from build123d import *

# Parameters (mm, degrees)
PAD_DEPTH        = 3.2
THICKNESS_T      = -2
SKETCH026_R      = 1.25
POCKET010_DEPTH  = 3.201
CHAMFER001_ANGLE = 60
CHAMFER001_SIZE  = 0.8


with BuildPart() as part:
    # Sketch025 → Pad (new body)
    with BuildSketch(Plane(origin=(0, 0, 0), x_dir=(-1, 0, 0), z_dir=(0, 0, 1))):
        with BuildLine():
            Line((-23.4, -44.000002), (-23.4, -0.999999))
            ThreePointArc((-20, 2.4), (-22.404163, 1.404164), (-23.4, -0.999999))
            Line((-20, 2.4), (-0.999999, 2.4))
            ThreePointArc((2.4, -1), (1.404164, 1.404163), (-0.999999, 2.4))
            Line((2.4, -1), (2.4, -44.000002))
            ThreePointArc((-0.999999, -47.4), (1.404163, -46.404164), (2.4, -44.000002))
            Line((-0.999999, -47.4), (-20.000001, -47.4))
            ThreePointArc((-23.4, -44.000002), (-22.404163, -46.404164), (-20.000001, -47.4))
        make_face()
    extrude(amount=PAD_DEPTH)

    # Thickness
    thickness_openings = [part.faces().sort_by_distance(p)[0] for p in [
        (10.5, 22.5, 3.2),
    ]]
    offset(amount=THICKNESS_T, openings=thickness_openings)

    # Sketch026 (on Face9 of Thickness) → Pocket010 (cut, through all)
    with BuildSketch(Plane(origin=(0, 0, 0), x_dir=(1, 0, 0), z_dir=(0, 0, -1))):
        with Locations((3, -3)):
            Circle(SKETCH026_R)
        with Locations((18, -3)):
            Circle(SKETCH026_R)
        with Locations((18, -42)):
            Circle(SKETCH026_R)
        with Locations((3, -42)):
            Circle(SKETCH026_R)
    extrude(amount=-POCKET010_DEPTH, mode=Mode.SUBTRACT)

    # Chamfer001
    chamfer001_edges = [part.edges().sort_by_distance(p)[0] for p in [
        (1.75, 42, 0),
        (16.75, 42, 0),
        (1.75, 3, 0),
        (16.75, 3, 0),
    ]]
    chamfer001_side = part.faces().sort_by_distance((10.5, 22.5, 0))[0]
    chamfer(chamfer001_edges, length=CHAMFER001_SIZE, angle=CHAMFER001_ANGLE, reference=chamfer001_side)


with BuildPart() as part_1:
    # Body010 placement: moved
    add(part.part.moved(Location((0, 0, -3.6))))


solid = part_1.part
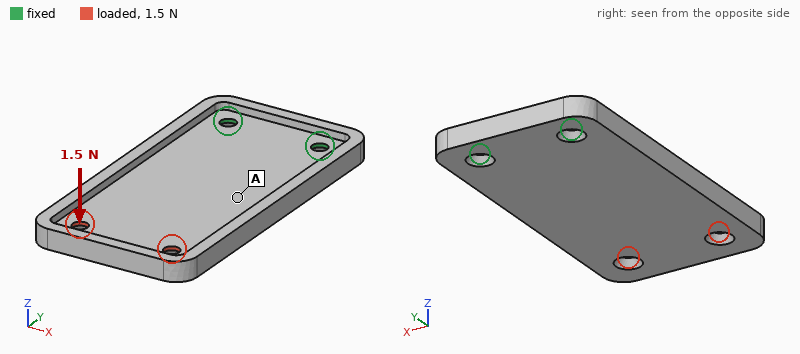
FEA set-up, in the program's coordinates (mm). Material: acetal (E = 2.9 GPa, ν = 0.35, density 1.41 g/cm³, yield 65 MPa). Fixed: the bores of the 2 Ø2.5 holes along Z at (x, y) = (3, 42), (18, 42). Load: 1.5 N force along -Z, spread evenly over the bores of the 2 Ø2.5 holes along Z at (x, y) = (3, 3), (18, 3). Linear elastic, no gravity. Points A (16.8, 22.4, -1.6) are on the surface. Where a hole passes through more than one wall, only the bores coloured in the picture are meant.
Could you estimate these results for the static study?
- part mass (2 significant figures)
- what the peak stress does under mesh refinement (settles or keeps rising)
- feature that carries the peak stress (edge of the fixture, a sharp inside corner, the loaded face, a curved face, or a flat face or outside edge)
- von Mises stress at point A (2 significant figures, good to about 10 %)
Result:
4.0 g
keeps rising
edge of the fixture
0.83 MPa
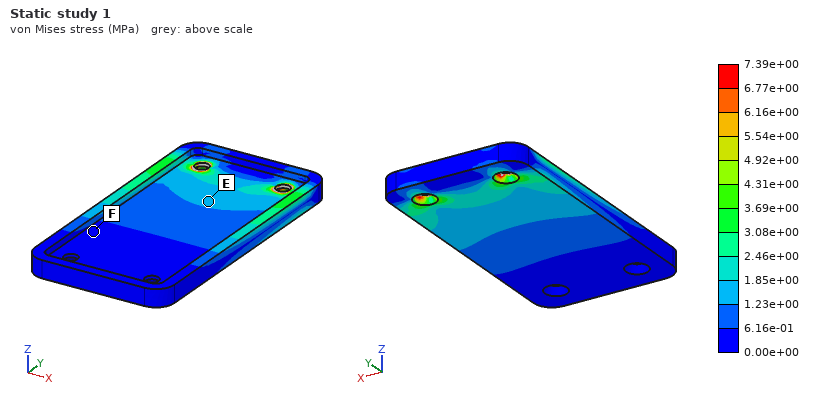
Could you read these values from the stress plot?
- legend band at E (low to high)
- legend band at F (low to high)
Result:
1.23e+00 to 1.85e+00 MPa
0.00e+00 to 6.16e-01 MPa
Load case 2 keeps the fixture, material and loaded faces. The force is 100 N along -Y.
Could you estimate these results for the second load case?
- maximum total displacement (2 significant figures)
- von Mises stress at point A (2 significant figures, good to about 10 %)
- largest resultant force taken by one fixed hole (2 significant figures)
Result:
0.64 mm
3.4 MPa
50 N
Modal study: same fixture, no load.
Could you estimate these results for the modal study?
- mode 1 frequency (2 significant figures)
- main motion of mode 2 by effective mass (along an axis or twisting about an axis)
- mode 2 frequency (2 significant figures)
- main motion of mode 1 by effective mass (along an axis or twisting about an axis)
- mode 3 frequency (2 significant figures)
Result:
220 Hz
twisting about Y
810 Hz
along Z
1500 Hz
